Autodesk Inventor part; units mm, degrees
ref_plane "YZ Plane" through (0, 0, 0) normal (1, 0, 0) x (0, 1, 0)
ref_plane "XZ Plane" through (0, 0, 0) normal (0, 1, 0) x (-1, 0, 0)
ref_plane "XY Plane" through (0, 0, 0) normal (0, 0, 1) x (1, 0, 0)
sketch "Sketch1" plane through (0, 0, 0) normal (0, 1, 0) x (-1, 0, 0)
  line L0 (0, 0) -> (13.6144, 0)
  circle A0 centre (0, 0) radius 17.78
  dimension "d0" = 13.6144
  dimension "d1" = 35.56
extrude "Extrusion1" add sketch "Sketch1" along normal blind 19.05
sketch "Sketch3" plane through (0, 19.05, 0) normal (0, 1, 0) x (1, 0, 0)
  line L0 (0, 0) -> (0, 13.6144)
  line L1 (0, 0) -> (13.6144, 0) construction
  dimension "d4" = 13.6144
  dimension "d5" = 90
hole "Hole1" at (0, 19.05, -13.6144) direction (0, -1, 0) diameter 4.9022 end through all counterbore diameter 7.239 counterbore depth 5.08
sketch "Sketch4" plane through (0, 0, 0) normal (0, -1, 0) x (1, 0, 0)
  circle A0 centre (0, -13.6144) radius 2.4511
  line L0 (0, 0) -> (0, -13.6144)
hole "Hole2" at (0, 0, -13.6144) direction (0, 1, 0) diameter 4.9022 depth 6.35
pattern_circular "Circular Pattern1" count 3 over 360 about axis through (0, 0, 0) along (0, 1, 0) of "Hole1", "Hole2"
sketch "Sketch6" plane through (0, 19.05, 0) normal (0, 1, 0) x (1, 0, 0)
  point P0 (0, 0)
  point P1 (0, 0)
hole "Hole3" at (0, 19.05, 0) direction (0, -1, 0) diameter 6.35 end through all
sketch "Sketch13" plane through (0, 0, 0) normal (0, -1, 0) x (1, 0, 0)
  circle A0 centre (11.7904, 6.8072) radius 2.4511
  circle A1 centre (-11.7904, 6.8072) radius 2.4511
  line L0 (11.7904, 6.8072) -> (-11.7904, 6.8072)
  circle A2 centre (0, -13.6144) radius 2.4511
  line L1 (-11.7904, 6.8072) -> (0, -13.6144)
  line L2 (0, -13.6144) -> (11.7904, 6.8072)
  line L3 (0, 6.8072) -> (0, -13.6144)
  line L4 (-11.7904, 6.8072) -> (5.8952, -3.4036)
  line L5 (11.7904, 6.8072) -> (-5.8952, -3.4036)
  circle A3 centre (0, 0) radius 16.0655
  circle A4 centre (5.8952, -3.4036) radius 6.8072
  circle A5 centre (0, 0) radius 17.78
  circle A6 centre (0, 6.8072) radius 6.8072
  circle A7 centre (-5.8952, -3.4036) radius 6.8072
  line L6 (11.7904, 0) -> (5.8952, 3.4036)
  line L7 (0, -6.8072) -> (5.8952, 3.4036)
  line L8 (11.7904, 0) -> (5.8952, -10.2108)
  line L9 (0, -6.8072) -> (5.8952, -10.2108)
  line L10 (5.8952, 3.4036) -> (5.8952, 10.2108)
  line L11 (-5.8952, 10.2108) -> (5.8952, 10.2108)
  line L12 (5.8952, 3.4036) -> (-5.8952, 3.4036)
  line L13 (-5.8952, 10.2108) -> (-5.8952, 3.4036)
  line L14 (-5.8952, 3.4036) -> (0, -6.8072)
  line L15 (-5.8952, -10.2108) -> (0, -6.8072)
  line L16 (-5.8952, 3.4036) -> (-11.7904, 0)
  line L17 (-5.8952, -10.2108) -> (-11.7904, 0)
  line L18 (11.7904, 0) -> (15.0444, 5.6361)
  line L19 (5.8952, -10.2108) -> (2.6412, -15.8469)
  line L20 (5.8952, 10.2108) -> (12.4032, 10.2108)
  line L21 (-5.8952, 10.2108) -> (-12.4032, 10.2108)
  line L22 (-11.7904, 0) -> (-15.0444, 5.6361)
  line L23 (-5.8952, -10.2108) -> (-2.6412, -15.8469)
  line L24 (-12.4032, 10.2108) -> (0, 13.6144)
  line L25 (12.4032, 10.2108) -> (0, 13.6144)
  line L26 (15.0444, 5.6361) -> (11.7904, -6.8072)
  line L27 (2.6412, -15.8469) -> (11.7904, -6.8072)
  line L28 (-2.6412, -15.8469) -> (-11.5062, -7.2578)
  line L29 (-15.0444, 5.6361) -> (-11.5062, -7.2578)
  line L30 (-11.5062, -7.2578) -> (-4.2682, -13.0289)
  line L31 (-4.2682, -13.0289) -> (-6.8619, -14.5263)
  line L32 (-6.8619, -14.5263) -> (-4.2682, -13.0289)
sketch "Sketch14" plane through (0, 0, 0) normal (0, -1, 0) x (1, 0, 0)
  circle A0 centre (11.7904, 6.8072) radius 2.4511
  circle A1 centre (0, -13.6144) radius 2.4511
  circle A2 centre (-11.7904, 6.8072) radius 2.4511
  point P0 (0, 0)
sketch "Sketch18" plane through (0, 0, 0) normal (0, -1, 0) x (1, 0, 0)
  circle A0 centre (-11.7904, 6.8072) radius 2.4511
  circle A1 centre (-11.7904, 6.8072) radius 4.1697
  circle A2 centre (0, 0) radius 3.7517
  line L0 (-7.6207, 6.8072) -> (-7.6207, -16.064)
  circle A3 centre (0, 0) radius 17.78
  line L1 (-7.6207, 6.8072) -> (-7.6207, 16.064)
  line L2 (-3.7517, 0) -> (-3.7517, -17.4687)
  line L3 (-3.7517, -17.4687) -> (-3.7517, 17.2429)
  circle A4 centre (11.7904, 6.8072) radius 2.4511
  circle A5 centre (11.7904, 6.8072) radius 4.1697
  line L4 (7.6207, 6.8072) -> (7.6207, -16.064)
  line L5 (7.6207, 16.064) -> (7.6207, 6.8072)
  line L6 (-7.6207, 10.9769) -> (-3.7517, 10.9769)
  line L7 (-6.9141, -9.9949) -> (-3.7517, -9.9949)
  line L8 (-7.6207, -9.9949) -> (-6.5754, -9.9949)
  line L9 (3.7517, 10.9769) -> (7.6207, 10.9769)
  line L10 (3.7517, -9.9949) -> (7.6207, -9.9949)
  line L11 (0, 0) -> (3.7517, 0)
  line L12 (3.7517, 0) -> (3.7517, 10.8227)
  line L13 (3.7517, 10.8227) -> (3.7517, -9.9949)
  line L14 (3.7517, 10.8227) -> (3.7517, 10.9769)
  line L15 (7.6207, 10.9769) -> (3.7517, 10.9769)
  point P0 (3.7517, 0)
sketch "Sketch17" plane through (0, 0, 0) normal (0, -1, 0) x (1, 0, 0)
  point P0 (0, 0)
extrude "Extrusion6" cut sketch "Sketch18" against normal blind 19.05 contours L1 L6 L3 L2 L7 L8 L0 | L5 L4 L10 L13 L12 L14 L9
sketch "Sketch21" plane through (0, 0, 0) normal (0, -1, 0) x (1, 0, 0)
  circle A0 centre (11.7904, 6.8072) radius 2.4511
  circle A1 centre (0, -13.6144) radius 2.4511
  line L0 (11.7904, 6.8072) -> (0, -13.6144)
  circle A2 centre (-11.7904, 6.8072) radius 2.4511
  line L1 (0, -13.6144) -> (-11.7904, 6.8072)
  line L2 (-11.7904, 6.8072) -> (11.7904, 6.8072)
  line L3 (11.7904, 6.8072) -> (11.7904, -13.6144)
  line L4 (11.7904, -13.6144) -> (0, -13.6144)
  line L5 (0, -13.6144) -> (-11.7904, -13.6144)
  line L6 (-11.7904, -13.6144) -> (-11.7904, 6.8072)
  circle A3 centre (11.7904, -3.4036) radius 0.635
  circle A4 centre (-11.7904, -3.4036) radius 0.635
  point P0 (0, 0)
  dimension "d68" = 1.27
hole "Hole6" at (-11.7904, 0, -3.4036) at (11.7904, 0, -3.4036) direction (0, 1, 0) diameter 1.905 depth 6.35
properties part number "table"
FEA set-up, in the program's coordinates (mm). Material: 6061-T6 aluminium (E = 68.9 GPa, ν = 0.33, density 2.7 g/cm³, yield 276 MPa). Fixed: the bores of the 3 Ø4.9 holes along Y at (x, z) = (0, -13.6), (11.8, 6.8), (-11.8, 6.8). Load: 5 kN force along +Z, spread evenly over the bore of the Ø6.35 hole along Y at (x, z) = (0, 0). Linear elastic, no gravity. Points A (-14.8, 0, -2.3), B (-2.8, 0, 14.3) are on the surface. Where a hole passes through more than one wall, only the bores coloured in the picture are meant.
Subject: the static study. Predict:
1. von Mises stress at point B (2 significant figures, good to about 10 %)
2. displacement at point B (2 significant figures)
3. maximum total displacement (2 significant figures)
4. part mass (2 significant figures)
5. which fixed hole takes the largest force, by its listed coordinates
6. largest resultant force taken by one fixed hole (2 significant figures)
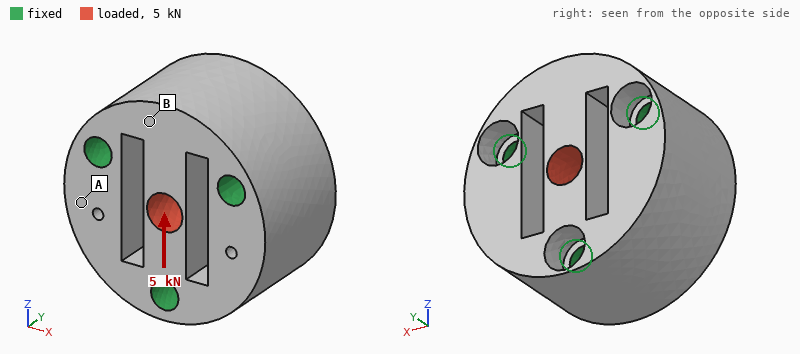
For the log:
17 MPa
4.7 µm
7.6 µm
37 g
(0, -13.6)
2.9 kN
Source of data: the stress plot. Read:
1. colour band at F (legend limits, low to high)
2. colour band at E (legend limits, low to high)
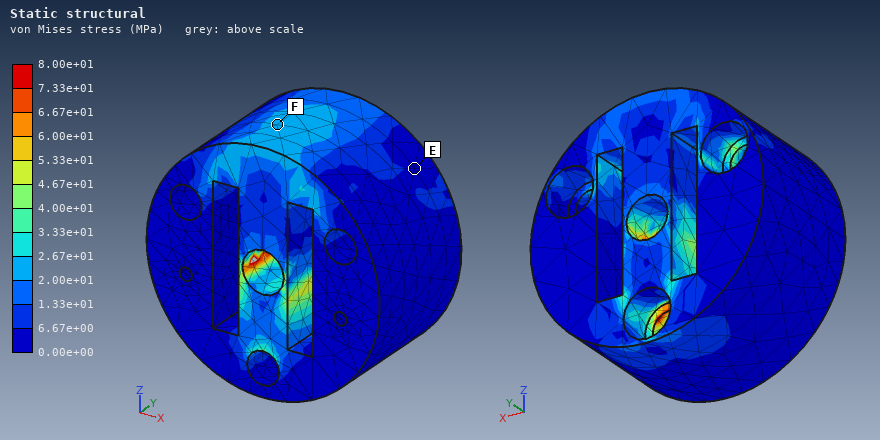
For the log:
2.00e+01 to 2.67e+01 MPa
0.00e+00 to 6.67e+00 MPa
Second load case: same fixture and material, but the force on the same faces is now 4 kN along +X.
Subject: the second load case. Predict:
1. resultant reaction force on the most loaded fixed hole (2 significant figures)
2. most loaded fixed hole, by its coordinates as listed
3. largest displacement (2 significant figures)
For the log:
2.1 kN
(0, -13.6)
24 µm
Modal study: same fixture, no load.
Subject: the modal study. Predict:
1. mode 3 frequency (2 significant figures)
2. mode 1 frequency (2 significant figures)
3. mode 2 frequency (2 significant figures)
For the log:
36 kHz
33 kHz
33 kHz
